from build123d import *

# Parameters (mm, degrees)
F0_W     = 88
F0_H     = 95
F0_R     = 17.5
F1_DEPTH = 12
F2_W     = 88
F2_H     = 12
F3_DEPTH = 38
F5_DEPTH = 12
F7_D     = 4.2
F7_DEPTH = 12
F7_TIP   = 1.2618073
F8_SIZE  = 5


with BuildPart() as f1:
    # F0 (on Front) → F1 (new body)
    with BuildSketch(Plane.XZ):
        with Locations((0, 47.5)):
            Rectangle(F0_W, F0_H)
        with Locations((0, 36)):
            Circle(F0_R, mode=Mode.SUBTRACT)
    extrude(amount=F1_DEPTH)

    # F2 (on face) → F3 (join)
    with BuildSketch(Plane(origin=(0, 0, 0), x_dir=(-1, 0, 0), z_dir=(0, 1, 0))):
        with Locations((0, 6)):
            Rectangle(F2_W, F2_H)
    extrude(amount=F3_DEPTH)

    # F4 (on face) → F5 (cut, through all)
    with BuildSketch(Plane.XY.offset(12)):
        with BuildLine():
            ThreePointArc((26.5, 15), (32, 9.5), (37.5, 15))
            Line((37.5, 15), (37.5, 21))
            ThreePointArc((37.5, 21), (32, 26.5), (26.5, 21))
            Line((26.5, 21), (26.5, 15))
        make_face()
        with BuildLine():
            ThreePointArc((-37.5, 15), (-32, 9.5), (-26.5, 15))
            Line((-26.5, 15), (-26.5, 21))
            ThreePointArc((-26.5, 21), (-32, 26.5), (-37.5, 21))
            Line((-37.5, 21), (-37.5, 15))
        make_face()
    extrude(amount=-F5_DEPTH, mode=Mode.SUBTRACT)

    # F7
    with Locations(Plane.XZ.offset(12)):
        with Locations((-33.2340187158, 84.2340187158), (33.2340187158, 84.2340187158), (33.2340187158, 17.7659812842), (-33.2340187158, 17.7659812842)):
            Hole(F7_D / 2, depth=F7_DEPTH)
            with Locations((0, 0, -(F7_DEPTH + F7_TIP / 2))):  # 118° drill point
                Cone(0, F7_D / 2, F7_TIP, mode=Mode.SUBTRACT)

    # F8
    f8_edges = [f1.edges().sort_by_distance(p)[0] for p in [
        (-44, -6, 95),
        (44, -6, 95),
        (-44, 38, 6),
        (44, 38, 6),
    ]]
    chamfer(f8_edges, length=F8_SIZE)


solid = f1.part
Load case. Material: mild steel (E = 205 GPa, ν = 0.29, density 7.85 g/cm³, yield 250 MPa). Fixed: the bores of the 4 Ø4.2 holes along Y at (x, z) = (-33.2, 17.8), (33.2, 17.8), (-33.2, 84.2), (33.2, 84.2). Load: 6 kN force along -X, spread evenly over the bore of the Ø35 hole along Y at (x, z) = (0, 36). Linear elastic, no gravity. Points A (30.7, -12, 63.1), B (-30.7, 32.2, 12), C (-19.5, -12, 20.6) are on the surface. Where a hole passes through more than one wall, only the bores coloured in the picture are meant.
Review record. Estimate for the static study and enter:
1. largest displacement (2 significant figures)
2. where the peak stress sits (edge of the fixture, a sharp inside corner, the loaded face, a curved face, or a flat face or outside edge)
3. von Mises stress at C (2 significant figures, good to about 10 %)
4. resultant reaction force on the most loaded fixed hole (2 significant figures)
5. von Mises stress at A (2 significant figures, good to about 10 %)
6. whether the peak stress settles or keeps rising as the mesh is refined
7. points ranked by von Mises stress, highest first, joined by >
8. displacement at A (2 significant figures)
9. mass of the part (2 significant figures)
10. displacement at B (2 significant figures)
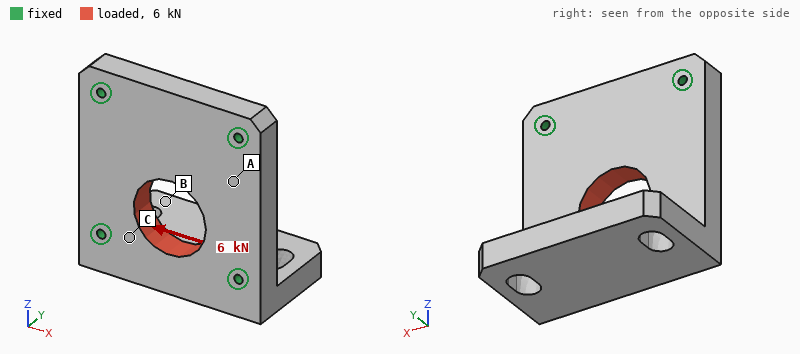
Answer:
1.5 µm
edge of the fixture
6.8 MPa
1.9 kN
3.6 MPa
keeps rising
C > A > B
0.91 µm
970 g
0.36 µm
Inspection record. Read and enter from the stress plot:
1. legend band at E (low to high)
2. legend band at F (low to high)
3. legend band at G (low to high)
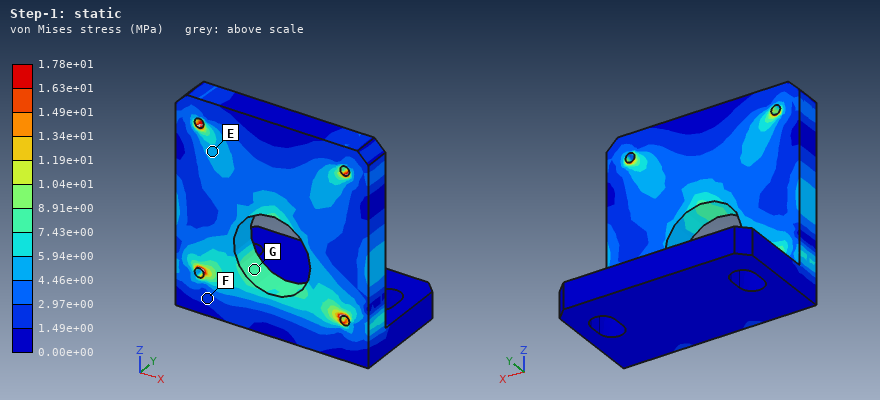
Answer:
4.46e+00 to 5.94e+00 MPa
1.49e+00 to 2.97e+00 MPa
7.43e+00 to 8.91e+00 MPa
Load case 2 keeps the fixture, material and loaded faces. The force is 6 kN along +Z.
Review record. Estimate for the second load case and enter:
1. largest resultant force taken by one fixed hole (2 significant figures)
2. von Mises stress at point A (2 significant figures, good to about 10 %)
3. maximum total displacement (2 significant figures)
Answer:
1.8 kN
3.5 MPa
2.2 µm
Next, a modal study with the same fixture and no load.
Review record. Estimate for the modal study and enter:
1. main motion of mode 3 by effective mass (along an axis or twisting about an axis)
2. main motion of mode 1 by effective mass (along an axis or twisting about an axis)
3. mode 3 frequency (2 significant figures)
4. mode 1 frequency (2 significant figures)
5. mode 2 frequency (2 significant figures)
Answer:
along Y
along Z
8300 Hz
3100 Hz
6100 Hz
